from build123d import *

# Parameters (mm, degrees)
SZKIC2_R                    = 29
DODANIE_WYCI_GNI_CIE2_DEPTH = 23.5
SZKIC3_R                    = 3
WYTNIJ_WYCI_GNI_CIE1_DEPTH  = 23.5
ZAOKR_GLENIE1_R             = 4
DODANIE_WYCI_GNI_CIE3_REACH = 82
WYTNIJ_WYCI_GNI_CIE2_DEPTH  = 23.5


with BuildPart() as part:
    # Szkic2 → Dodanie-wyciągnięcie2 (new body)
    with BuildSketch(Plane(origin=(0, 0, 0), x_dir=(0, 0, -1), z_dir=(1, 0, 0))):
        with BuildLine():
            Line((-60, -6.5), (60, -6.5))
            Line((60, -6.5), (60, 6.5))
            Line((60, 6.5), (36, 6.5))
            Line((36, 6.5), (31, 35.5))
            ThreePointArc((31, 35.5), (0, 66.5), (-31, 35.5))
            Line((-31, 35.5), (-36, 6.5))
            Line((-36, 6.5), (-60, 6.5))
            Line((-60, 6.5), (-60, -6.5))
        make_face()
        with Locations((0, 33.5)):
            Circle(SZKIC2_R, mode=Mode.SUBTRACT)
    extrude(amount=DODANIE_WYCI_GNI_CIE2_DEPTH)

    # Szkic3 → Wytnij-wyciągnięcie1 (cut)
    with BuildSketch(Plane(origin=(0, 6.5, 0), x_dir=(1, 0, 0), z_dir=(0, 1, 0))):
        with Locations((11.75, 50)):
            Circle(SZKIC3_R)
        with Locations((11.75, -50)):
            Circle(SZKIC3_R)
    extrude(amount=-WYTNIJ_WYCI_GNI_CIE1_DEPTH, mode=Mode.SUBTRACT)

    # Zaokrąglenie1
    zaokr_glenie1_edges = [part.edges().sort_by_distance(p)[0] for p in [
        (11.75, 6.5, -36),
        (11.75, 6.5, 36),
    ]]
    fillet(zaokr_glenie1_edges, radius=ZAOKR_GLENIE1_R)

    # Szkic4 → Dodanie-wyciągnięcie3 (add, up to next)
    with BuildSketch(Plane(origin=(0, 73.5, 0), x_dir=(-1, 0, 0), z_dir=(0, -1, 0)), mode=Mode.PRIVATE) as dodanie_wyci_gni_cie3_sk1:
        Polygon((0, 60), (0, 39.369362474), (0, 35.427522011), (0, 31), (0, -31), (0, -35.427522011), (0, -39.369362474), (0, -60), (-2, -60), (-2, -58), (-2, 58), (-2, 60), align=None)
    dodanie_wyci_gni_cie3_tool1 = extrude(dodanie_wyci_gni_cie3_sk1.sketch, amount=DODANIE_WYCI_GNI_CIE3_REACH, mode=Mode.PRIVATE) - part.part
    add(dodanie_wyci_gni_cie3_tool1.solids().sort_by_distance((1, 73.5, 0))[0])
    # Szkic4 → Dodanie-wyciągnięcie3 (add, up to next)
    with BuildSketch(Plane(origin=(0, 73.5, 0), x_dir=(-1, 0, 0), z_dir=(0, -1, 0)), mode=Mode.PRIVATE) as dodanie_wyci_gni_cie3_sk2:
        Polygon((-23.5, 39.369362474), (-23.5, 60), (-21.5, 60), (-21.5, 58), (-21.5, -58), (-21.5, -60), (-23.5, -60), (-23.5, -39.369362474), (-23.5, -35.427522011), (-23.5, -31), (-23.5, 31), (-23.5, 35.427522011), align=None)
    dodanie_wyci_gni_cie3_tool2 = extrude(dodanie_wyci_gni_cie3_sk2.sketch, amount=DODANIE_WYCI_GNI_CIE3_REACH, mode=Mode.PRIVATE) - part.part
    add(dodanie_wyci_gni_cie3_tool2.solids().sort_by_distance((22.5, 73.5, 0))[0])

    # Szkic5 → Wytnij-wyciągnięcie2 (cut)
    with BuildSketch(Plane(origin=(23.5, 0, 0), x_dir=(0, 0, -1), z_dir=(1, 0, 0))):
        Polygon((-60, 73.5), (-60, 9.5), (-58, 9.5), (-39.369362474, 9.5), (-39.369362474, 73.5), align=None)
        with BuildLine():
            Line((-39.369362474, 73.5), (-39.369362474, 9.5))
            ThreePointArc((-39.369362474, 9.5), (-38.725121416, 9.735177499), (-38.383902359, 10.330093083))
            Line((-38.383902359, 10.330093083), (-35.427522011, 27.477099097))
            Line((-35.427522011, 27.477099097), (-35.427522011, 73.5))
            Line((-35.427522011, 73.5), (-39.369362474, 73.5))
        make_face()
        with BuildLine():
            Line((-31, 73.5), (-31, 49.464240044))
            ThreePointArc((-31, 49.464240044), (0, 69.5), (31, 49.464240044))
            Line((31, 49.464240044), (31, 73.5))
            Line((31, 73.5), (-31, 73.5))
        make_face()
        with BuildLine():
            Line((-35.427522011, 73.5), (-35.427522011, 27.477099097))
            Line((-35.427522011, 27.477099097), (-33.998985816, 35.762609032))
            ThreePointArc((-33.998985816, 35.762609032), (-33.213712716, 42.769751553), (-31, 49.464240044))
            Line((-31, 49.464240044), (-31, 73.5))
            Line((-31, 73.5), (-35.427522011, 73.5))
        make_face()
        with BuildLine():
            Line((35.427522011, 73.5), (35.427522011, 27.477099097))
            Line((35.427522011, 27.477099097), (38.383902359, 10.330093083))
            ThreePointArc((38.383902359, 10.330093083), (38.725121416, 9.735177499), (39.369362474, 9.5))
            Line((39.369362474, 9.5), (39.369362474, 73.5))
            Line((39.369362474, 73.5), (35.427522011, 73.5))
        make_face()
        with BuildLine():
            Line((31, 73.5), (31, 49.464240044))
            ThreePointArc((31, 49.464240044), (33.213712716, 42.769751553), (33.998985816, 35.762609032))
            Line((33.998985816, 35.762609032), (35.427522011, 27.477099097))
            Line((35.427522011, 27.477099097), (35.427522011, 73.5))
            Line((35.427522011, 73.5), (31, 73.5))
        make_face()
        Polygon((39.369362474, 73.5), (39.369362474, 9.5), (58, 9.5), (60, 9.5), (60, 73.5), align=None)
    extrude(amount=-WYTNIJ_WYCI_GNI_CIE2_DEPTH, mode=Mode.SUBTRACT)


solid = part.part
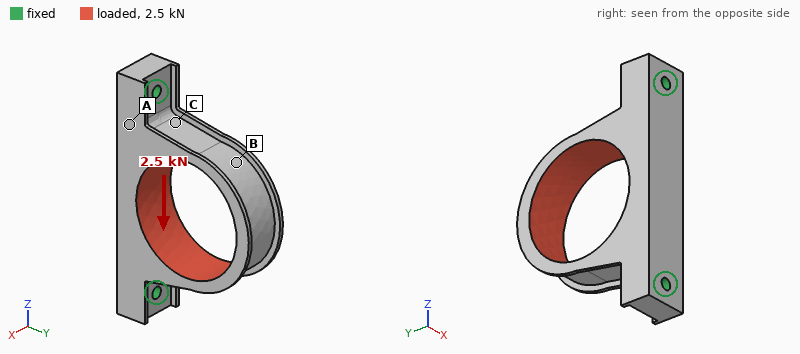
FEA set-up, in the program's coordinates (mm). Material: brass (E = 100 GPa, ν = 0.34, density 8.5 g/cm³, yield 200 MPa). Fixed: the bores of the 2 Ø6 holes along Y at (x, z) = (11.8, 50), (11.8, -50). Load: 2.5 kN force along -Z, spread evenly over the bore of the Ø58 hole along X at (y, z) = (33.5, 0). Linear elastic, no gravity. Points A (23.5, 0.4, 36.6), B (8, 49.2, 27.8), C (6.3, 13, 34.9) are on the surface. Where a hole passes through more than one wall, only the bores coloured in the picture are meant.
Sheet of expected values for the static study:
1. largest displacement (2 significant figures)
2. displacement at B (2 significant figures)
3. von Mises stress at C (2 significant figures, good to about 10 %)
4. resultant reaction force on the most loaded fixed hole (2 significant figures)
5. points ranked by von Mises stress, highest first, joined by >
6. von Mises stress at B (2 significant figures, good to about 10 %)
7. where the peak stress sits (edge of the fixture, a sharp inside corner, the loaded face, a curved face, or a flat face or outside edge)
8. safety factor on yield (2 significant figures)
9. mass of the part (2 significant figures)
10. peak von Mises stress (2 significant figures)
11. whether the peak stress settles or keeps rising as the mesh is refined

0.14 mm
0.12 mm
24 MPa
1.5 kN
B > C > A
39 MPa
a flat face or outside edge
1.6
490 g
120 MPa
settles
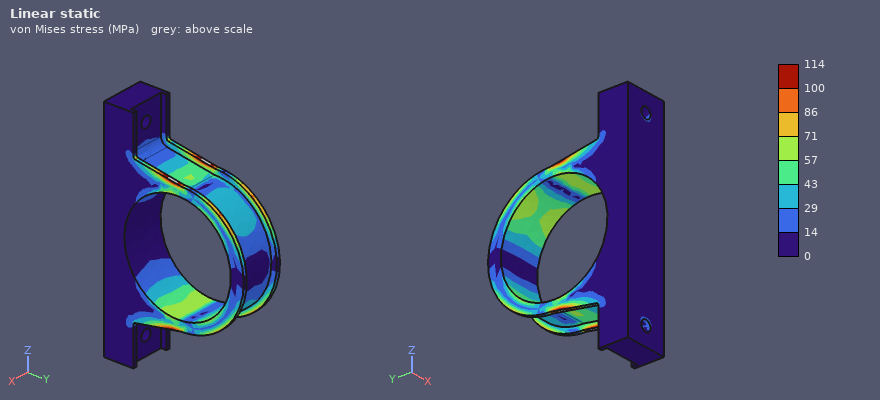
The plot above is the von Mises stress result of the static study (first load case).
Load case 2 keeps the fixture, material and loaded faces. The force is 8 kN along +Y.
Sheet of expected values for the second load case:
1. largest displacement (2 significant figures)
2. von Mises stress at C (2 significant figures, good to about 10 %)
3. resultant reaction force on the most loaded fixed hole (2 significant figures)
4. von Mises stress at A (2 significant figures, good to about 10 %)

58 µm
32 MPa
4.0 kN
26 MPa
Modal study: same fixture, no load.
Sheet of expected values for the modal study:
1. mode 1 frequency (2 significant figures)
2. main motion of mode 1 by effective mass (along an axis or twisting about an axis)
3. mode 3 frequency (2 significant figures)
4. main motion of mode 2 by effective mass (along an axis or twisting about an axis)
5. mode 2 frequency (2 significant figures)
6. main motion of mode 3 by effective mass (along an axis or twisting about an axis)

1700 Hz
along X
3300 Hz
along Z
1900 Hz
along Y
